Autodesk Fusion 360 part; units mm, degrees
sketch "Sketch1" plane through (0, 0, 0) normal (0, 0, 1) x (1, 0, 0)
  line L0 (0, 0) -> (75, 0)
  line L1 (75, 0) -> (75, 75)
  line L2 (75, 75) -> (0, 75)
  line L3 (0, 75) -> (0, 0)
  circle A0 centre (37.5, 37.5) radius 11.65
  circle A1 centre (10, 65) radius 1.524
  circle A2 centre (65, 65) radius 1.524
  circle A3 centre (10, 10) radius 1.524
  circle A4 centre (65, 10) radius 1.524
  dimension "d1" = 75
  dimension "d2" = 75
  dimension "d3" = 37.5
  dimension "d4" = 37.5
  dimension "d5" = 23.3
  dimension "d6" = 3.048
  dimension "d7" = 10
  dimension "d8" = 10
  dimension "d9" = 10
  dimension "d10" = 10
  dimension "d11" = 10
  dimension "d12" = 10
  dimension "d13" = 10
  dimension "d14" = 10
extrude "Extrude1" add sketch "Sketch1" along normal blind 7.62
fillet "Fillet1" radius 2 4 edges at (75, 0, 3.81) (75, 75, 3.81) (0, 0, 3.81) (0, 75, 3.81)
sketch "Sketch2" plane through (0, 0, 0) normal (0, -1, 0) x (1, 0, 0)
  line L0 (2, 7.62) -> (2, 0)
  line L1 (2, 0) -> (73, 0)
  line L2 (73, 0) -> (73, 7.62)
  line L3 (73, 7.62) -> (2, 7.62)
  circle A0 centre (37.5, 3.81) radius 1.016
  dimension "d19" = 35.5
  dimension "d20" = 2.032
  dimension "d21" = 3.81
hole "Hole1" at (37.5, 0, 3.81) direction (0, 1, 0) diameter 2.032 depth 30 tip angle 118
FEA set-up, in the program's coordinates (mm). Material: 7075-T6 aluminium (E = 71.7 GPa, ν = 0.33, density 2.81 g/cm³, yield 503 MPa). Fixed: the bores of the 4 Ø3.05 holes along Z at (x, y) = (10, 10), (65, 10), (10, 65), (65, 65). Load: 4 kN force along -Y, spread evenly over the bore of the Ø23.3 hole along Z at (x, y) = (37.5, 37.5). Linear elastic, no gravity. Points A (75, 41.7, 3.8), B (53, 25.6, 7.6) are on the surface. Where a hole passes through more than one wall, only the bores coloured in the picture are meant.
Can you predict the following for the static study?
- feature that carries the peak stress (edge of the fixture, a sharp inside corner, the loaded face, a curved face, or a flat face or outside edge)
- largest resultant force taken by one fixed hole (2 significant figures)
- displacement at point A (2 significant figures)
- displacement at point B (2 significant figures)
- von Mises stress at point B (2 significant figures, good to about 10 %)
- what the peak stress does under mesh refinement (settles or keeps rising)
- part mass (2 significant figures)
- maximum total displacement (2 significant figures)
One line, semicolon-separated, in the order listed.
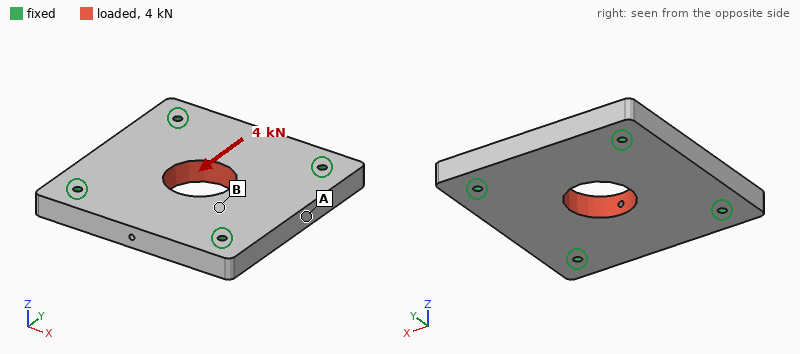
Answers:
edge of the fixture; 1.1 kN; 1.1 µm; 2.9 µm; 7.0 MPa; keeps rising; 110 g; 4.9 µm
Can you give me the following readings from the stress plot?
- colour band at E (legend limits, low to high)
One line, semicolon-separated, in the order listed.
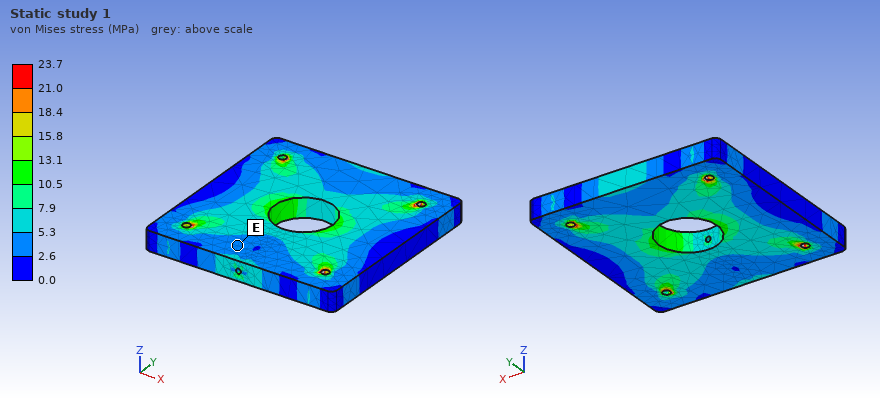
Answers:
2.6 to 5.3 MPa
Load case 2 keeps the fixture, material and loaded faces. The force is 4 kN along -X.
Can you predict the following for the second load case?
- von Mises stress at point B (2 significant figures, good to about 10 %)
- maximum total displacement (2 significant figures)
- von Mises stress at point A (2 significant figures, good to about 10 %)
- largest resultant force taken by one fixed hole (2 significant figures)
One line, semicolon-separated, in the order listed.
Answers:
7.0 MPa; 4.9 µm; 6.6 MPa; 1.1 kN
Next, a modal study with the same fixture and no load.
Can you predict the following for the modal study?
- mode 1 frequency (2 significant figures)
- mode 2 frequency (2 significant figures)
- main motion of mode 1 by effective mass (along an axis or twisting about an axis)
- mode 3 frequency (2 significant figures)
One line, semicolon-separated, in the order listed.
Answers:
7900 Hz; 11 kHz; along Z; 11 kHz
